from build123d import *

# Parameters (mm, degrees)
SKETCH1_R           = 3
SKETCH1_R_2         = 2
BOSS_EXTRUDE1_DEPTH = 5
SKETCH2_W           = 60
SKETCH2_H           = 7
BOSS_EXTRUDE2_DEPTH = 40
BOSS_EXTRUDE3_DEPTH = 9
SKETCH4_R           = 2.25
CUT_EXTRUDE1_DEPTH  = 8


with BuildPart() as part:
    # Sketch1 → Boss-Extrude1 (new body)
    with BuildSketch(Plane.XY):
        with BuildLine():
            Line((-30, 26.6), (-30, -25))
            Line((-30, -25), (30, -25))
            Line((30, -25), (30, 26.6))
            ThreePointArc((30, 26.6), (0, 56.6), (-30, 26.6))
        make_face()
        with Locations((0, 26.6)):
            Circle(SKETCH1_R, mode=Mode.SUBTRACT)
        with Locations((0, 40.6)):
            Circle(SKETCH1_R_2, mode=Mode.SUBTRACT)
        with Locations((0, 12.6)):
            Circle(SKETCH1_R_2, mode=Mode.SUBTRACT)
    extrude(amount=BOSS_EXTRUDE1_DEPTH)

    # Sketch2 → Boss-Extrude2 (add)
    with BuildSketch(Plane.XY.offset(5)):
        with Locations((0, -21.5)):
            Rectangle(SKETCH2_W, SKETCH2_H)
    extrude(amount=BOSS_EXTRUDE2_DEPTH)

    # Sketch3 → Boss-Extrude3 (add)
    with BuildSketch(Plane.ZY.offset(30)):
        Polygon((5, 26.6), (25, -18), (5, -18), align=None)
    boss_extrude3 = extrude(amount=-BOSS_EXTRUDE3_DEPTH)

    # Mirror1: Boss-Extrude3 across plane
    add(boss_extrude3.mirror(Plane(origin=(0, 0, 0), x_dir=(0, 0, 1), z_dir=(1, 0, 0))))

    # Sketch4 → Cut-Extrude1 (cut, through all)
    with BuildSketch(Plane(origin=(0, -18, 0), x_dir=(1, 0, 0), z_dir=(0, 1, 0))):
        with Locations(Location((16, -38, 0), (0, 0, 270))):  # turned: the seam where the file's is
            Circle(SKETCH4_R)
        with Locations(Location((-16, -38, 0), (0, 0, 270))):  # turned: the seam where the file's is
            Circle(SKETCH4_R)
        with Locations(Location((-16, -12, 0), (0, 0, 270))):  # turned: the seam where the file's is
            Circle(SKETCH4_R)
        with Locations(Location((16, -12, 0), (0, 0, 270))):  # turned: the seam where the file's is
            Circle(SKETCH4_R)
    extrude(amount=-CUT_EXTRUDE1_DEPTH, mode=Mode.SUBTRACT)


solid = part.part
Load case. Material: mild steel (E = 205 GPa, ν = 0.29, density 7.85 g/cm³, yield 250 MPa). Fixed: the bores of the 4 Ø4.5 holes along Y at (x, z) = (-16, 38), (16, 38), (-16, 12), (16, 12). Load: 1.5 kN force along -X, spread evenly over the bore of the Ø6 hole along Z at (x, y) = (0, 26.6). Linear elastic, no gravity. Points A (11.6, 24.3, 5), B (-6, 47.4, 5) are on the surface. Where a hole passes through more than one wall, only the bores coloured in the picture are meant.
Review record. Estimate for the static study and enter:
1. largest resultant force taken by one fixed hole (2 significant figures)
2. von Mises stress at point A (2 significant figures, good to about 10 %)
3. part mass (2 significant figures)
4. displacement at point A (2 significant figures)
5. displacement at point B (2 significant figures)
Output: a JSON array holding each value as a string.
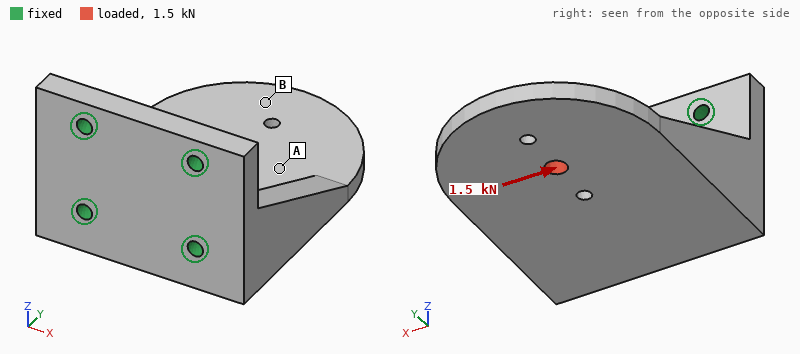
["2.1 kN", "16 MPa", "370 g", "16 µm", "22 µm"]
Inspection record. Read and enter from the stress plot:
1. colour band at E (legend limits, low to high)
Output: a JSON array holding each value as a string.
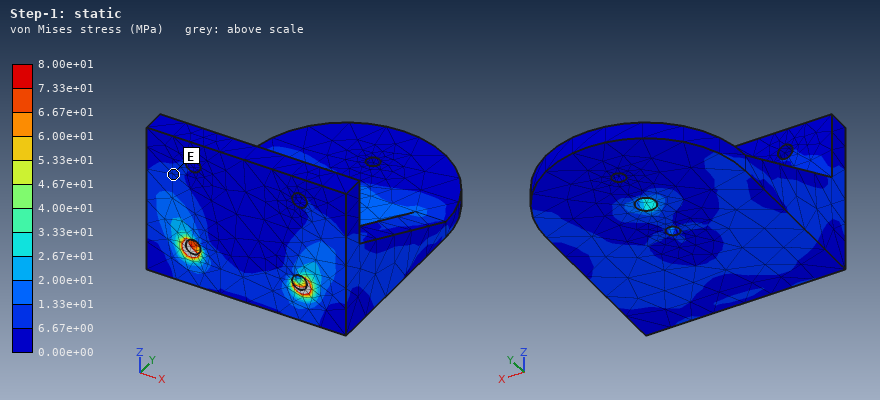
["6.67e+00 to 1.33e+01 MPa"]
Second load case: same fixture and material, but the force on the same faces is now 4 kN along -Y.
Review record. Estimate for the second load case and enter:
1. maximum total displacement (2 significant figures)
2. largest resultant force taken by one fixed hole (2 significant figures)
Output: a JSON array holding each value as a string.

["34 µm", "2.4 kN"]
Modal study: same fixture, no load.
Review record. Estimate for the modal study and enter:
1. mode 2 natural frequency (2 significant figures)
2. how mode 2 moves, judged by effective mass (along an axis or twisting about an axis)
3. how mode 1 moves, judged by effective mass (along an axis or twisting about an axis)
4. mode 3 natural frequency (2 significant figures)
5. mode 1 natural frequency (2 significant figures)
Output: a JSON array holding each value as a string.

["3500 Hz", "along X", "along Z", "5700 Hz", "2000 Hz"]
